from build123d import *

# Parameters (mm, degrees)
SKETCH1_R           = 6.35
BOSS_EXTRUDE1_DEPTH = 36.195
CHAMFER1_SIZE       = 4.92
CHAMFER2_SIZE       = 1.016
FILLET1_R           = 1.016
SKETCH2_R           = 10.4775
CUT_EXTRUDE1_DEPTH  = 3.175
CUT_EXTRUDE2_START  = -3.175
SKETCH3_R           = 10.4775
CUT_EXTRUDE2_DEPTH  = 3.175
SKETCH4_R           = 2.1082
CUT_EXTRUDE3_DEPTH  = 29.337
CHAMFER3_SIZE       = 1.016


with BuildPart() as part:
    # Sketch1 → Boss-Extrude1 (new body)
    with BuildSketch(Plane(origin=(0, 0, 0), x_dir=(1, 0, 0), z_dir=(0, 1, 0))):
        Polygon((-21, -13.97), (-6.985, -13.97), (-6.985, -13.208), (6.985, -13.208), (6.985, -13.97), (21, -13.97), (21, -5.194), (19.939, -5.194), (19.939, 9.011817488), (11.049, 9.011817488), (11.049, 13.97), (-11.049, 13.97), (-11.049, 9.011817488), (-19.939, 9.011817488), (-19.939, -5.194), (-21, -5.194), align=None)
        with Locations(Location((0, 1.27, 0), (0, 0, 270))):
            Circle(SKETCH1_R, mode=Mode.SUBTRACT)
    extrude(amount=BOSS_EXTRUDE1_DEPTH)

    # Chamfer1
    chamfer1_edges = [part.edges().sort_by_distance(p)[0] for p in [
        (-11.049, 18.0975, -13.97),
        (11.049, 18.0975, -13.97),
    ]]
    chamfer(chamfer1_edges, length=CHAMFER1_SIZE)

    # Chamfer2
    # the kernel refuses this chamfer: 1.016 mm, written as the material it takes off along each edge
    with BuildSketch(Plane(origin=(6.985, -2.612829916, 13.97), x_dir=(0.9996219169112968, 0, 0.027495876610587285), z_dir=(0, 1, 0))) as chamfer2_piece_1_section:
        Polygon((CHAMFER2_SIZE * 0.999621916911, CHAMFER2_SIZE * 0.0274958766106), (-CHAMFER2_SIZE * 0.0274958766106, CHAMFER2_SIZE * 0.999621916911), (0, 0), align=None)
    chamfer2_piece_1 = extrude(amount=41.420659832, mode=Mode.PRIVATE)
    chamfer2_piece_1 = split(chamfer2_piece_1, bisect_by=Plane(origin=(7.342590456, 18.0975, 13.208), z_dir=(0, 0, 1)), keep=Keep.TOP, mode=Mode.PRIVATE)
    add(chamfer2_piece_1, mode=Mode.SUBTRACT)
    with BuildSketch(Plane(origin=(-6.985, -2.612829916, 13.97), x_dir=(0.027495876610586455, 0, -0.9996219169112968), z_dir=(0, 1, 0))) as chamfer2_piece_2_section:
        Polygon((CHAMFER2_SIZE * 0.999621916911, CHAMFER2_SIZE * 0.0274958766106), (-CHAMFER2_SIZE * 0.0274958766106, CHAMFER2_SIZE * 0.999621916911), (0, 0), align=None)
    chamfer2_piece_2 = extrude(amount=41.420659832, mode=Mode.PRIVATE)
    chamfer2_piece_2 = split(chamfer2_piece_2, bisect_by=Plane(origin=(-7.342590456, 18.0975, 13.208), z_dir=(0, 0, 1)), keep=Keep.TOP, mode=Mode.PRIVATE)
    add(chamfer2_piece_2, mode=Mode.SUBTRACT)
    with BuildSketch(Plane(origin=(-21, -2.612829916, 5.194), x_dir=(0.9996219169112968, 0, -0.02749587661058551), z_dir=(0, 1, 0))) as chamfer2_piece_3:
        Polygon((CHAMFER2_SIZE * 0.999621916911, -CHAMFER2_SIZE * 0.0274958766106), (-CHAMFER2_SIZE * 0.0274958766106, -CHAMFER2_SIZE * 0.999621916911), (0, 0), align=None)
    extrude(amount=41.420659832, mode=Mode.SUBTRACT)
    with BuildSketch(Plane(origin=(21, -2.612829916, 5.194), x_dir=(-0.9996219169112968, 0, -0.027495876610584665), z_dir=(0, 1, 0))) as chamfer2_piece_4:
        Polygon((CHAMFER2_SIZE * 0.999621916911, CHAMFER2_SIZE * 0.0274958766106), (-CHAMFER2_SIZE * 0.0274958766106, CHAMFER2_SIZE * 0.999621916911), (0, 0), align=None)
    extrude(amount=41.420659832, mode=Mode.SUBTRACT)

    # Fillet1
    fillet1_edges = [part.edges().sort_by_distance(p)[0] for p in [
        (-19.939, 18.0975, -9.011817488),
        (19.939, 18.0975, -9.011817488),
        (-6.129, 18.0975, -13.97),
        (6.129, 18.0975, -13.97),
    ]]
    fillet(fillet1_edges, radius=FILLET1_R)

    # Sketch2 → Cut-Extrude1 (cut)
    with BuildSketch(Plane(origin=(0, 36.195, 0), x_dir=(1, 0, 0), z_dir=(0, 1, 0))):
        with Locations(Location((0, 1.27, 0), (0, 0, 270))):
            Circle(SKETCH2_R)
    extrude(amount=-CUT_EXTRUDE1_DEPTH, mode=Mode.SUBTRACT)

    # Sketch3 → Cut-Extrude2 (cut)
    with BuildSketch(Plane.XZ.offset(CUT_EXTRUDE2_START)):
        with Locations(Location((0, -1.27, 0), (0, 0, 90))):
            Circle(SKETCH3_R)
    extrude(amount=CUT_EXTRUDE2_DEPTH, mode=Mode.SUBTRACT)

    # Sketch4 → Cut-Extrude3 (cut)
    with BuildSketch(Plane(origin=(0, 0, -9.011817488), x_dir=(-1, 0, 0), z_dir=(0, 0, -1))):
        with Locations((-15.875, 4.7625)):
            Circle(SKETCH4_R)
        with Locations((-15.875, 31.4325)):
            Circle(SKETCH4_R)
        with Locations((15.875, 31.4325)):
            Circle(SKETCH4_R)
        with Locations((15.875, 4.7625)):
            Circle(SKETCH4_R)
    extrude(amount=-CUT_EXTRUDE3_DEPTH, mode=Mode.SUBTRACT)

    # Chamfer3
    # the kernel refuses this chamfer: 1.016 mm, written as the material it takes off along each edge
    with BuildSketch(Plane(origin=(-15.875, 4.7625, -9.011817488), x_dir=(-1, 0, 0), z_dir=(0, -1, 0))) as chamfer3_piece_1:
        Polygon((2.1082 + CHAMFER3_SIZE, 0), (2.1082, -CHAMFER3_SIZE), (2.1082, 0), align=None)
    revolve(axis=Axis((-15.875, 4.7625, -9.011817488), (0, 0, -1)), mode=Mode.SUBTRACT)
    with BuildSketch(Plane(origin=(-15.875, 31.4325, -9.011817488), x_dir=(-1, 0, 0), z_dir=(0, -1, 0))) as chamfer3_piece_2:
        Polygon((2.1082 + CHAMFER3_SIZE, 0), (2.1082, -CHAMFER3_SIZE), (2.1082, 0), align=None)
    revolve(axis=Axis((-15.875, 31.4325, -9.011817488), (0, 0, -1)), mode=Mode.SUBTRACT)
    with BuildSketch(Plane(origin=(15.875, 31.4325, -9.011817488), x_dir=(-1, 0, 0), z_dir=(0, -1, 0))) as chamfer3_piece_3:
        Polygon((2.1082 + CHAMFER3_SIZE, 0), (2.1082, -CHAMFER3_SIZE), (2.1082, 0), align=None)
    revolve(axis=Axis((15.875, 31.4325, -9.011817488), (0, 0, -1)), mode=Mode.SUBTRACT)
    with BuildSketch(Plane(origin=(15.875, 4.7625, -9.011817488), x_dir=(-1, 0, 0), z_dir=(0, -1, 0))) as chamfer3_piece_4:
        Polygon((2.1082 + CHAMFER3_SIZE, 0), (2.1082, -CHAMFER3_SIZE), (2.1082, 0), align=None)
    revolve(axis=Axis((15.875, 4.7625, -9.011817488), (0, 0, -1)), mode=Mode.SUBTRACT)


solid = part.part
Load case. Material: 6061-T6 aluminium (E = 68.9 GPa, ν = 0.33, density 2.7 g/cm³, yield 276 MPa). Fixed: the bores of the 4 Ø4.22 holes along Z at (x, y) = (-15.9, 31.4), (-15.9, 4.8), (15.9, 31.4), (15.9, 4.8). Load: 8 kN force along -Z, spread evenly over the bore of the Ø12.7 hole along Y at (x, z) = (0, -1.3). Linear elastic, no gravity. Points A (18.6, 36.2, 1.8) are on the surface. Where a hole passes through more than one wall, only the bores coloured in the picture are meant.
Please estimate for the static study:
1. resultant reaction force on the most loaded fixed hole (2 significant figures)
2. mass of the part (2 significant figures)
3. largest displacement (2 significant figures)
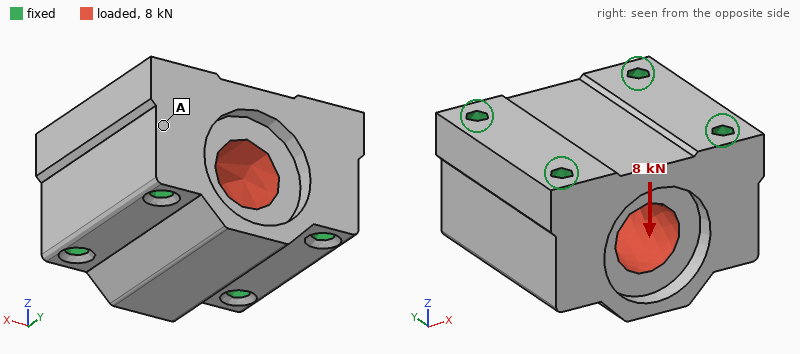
2.0 kN
79 g
4.8 µm
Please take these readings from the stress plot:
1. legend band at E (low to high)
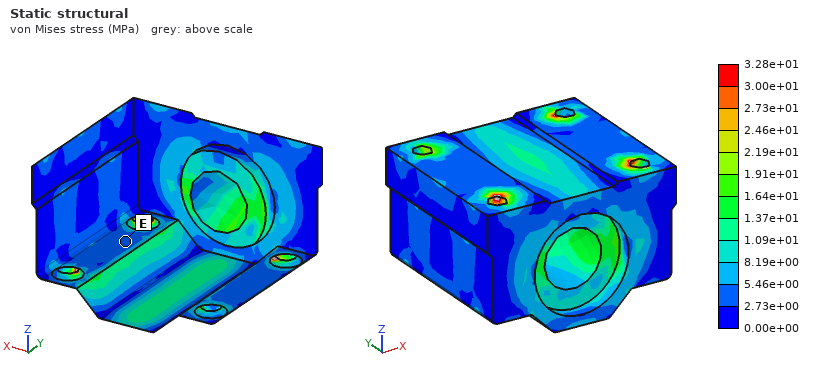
2.73e+00 to 5.46e+00 MPa
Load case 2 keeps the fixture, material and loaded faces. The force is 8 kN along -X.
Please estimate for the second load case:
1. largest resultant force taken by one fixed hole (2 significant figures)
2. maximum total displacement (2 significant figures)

2.1 kN
3.1 µm
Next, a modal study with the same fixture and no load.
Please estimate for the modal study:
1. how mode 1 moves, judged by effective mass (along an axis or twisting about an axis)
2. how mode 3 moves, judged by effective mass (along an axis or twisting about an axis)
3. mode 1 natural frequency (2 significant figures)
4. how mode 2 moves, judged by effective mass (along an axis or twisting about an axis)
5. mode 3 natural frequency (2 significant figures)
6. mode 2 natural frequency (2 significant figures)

along Z
along X
39 kHz
along Y
46 kHz
41 kHz
